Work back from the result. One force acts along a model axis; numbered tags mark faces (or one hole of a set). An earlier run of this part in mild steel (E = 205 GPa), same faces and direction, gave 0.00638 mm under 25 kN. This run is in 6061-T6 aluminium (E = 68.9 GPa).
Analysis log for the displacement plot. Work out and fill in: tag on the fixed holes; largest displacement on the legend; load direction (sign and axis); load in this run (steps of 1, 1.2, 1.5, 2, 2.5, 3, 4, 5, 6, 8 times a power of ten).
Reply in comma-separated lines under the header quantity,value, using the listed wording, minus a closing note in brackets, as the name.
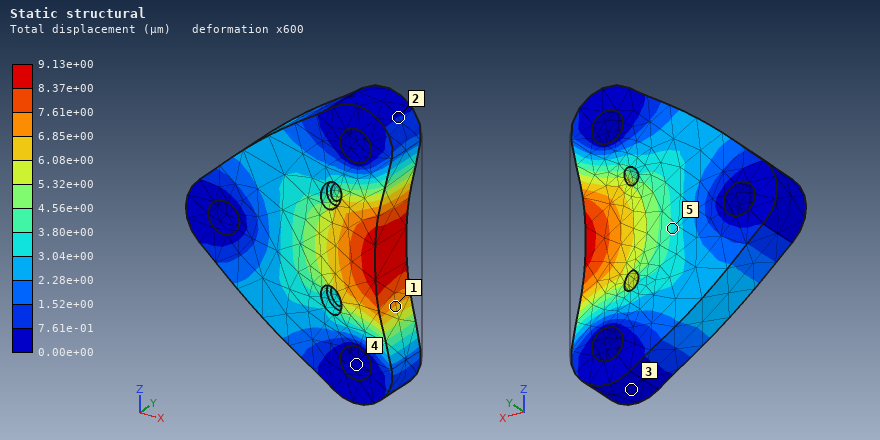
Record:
quantity,value
tag on the fixed holes,4
largest displacement on the legend,9.13e+00 µm
load direction,-X
load in this run,12 kN
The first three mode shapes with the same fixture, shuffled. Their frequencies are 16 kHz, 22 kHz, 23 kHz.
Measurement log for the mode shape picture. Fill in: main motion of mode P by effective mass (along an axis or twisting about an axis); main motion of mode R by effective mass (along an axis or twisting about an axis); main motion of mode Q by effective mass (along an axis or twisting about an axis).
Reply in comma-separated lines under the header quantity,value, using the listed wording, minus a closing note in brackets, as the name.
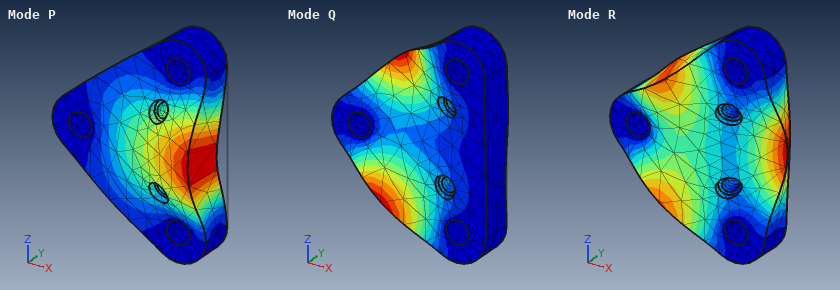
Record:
quantity,value
main motion of mode P by effective mass,along Y
main motion of mode R by effective mass,along Y
main motion of mode Q by effective mass,twisting about X
